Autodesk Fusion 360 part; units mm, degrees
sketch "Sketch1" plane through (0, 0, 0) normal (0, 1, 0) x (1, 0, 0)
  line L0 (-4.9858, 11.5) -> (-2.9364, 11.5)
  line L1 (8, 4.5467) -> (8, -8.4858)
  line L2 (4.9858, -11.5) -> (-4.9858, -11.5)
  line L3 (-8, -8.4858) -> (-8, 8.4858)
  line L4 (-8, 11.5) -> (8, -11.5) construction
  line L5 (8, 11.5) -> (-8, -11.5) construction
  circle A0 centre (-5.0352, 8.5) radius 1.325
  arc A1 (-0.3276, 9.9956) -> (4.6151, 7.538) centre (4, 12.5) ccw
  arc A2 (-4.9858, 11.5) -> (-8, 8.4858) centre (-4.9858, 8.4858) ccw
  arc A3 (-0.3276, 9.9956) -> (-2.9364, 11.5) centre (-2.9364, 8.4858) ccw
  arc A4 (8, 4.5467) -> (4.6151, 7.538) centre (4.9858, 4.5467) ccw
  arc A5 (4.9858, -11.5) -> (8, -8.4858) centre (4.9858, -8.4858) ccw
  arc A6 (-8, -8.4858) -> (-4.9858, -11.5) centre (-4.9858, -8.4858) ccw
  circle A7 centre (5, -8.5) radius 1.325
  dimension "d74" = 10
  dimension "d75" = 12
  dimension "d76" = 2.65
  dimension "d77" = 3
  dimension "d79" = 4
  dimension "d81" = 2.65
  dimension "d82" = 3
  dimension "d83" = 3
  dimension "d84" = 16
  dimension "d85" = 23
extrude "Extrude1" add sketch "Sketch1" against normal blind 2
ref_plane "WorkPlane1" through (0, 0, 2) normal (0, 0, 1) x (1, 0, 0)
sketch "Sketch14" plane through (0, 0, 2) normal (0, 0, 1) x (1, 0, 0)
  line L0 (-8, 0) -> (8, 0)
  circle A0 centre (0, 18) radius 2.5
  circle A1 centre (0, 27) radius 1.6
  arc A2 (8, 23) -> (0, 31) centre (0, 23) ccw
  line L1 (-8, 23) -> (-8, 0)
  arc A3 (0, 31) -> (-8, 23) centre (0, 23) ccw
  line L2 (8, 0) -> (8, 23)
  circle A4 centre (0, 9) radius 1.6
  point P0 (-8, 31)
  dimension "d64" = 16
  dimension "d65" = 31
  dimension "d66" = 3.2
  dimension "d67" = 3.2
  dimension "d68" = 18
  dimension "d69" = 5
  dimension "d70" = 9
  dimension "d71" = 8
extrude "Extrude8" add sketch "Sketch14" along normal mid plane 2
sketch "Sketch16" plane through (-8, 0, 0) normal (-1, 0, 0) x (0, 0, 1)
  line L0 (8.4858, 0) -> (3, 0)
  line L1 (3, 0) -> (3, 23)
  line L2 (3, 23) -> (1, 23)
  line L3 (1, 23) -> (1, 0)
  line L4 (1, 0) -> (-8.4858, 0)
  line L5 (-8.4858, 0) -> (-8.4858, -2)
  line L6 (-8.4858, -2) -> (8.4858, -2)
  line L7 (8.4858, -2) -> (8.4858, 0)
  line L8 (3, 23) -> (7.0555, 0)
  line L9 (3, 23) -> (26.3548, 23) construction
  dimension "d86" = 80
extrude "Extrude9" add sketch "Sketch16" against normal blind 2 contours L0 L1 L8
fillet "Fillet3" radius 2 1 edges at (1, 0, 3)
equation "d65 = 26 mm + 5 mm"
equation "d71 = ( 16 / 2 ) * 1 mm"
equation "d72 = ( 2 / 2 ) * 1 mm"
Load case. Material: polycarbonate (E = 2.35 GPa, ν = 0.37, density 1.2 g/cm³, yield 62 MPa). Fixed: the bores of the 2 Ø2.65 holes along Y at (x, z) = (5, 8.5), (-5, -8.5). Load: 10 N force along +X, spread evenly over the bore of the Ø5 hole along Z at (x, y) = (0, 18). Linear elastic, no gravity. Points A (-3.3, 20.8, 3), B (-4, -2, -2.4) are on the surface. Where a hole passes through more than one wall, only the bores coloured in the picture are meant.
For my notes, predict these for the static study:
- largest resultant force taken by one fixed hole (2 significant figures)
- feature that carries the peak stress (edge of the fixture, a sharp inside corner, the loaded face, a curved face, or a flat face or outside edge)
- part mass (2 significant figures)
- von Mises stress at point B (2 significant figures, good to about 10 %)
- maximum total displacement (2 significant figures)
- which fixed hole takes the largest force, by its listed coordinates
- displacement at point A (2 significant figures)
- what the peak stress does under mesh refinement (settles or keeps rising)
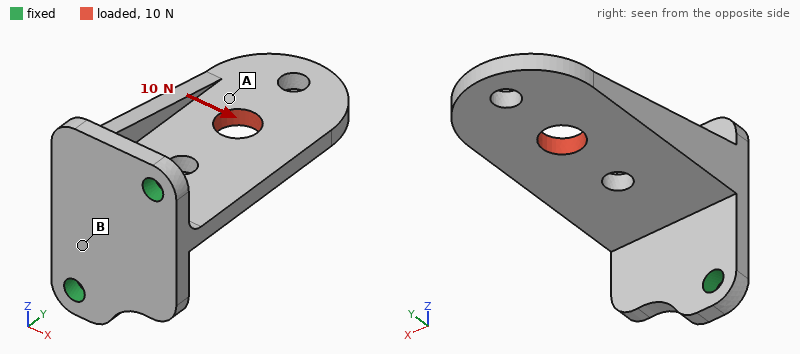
9.2 N
edge of the fixture
1.9 g
4.5 MPa
0.52 mm
(5, 8.5)
0.36 mm
keeps rising
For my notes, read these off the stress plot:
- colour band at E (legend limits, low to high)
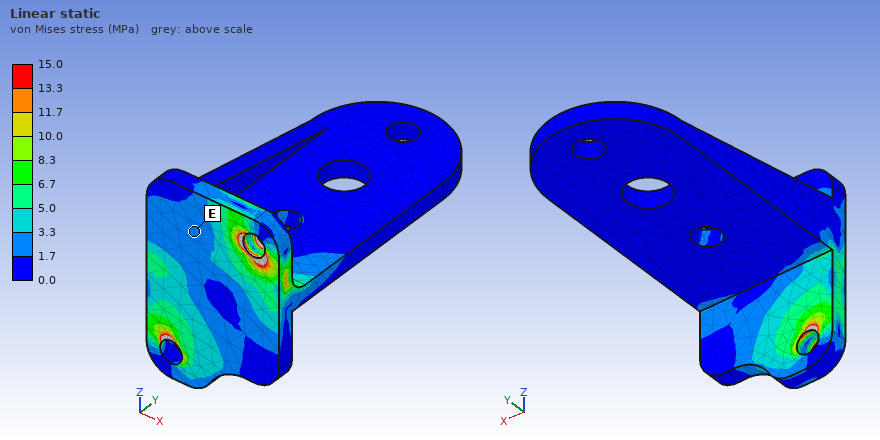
1.7 to 3.3 MPa
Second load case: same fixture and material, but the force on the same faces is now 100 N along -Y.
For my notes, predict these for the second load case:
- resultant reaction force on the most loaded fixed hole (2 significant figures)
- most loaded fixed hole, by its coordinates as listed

62 N
(5, 8.5)
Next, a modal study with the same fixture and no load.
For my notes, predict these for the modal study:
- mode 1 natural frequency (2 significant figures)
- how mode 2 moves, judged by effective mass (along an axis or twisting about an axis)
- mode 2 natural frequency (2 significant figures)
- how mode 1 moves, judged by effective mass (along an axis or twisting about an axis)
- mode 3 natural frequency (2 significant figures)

620 Hz
along X
970 Hz
along Z
2100 Hz
